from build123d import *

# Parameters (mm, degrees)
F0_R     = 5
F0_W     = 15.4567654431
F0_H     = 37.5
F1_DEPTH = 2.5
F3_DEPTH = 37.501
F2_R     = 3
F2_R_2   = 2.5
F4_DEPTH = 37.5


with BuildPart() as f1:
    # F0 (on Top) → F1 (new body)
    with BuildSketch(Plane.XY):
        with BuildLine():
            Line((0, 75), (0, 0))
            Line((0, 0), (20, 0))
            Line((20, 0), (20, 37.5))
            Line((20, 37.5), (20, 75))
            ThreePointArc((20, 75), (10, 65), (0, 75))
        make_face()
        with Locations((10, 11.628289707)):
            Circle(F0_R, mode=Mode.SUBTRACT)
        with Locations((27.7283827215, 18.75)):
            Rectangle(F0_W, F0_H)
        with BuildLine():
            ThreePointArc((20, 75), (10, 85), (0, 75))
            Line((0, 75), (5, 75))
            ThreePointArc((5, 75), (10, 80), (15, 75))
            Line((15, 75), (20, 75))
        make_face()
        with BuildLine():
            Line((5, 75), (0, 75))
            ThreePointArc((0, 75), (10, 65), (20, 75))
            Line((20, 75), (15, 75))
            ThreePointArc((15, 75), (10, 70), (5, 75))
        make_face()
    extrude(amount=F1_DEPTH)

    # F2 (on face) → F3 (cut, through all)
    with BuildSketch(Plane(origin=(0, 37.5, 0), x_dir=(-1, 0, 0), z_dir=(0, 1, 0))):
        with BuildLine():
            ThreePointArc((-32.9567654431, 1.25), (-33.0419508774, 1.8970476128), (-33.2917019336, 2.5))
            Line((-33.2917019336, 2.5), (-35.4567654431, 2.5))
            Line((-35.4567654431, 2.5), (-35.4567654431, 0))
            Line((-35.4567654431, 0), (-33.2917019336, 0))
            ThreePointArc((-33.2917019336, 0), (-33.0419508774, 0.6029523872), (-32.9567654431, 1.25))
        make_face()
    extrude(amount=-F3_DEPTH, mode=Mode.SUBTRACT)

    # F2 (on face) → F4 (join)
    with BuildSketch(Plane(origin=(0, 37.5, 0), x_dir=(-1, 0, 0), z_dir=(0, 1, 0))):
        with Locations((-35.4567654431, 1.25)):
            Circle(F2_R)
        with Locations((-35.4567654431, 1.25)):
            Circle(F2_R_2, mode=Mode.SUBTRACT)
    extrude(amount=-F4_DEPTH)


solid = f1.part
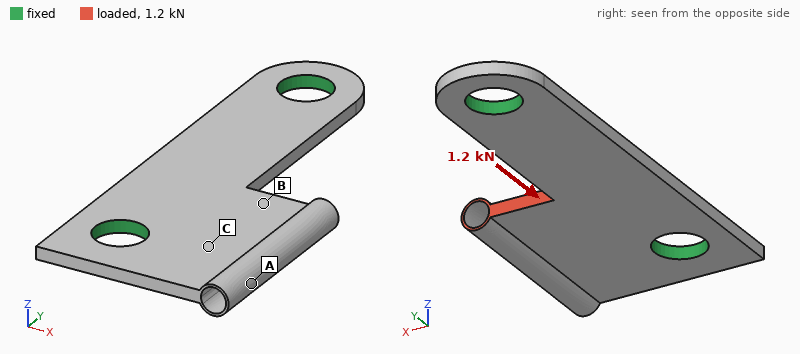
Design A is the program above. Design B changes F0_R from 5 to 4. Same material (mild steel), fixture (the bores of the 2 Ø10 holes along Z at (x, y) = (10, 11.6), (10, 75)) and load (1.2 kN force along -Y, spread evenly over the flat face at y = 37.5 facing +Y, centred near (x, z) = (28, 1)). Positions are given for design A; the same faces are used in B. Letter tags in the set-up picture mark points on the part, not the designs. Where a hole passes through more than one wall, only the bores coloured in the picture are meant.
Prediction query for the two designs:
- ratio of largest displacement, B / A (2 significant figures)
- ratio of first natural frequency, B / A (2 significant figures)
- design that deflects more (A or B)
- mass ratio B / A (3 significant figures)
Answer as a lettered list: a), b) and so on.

a) 1.1
b) 0.93
c) B
d) 1.01
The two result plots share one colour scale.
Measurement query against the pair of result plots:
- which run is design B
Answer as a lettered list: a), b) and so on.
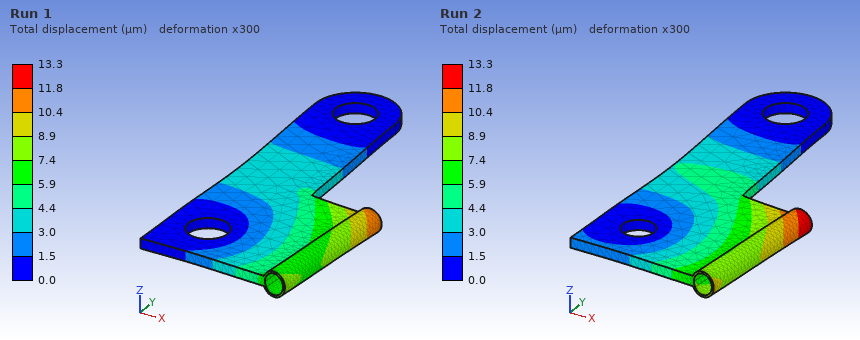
a) Run 2
